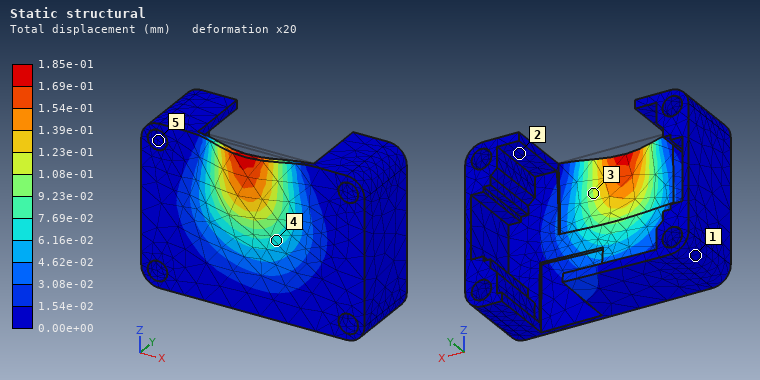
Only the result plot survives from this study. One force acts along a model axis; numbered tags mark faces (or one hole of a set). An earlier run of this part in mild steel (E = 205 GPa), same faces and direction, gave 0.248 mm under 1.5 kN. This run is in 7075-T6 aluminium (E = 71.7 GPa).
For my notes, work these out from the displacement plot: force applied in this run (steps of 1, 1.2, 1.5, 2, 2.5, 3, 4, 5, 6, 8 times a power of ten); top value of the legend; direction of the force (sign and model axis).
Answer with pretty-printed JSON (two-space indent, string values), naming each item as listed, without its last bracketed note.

{
  "force applied in this run": "400 N",
  "top value of the legend": "1.85e-01 mm",
  "direction of the force": "-Y"
}
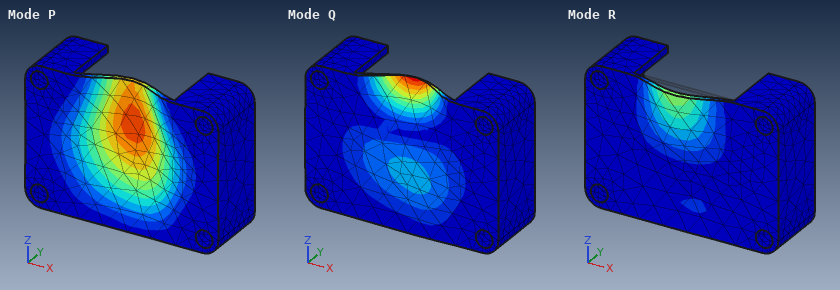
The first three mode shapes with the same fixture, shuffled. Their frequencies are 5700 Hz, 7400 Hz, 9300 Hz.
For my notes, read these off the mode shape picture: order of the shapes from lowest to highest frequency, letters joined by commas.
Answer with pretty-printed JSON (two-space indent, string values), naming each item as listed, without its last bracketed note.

{
  "order of the shapes from lowest to highest frequency, letters joined by commas": "P, R, Q"
}
